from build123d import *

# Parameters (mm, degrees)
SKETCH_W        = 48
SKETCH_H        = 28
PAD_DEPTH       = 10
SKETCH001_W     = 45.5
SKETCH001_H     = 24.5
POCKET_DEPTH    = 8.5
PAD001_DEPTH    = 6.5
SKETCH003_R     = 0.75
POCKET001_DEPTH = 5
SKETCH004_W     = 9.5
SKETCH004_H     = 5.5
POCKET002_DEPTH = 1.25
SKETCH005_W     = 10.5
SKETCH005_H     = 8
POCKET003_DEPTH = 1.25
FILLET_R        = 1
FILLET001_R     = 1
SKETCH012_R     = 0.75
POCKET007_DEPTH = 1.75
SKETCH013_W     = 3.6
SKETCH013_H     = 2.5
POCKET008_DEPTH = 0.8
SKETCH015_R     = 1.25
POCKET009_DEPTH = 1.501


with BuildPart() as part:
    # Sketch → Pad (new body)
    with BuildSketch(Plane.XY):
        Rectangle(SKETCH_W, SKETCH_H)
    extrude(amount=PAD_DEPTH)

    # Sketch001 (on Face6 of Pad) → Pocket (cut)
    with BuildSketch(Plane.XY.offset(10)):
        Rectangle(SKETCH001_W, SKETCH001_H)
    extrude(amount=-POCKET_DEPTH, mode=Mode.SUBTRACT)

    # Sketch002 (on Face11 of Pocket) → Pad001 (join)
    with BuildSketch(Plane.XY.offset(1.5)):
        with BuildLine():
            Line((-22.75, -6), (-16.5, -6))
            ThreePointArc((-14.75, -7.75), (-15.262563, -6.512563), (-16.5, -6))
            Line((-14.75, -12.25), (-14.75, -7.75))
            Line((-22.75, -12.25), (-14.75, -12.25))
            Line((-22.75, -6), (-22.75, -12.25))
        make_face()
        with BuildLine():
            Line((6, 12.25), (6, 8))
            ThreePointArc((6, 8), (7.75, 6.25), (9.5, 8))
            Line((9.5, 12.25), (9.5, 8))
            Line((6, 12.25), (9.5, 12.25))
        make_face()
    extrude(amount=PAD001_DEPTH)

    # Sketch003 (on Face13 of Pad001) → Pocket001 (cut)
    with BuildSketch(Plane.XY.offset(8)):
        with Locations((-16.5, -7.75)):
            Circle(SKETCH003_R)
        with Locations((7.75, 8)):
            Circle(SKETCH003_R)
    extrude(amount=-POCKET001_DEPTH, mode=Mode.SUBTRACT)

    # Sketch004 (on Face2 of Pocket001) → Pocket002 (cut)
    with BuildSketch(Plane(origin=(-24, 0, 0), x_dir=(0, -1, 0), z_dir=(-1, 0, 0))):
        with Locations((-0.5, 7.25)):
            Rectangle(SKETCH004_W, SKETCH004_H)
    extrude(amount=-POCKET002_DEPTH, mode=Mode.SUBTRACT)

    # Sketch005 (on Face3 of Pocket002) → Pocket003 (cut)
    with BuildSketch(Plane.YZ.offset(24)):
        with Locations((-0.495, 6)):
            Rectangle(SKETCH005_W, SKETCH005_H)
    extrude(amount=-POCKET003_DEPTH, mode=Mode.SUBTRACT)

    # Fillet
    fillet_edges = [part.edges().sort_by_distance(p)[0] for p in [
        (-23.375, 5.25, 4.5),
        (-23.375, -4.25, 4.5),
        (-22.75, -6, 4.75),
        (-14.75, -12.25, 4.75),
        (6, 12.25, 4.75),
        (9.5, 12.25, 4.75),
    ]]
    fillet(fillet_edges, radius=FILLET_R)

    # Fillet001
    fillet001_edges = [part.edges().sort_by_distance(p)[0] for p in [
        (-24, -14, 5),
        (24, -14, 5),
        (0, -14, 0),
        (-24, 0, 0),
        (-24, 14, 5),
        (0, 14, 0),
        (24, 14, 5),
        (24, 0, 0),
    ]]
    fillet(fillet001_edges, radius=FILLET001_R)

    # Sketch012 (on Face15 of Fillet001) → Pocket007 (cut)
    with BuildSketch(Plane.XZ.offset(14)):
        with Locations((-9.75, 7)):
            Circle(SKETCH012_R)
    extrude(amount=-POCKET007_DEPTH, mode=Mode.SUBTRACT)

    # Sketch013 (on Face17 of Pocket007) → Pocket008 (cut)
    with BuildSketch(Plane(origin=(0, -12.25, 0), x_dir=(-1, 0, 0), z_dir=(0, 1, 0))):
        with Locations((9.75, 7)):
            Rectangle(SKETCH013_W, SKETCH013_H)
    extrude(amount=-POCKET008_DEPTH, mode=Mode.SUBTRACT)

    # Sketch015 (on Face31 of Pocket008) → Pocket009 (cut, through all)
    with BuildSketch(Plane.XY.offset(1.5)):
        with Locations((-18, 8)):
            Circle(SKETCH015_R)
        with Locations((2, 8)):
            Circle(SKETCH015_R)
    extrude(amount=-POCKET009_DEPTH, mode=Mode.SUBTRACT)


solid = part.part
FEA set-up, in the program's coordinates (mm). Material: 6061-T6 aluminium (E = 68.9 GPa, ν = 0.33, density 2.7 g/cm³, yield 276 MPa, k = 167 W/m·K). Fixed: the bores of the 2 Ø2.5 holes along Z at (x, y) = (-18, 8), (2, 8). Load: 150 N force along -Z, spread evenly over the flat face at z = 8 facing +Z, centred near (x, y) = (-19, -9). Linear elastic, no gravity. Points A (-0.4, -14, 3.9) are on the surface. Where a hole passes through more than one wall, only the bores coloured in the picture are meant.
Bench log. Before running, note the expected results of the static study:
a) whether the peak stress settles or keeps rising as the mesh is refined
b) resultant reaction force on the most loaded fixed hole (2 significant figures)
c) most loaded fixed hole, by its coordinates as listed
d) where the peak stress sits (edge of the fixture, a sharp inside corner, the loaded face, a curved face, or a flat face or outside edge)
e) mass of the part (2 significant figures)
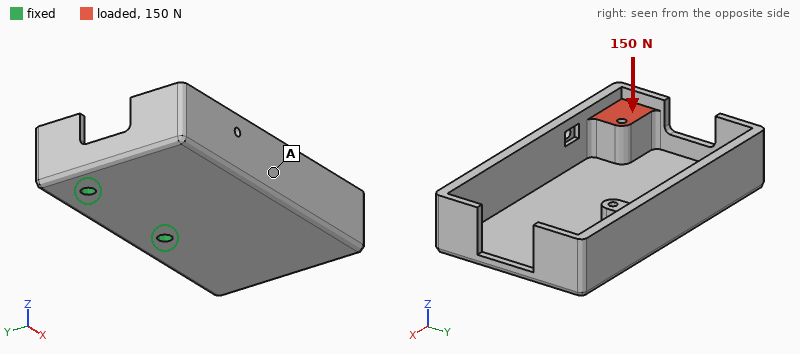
keeps rising
140 N
(-18, 8)
edge of the fixture
11 g
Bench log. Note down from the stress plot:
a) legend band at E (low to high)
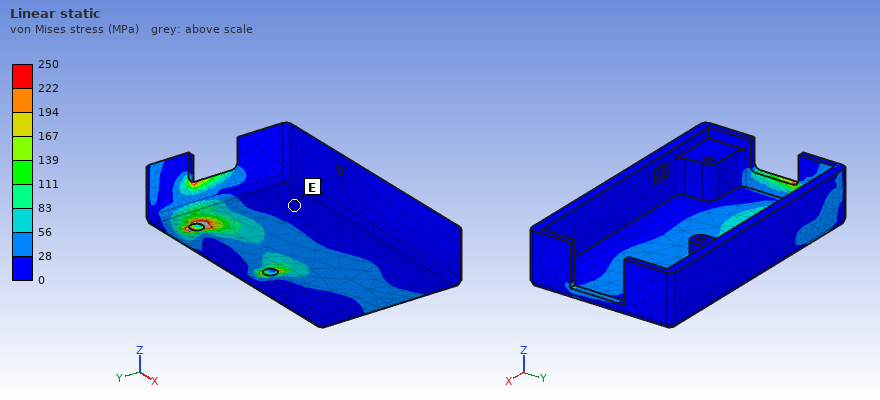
0 to 28 MPa
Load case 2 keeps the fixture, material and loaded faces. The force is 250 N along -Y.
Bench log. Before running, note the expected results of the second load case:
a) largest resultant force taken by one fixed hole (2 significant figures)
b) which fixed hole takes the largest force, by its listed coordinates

250 N
(-18, 8)
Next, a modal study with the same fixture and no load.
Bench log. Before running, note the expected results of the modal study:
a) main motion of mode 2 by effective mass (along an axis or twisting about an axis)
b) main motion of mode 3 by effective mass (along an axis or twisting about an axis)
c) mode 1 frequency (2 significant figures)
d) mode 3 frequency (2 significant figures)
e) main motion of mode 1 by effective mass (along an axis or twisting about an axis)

twisting about Y
along Z
1500 Hz
5500 Hz
along Z
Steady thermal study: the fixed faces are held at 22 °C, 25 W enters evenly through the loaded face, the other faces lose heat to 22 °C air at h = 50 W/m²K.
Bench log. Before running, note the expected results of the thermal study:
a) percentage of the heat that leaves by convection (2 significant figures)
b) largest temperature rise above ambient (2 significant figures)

21 %
70 K
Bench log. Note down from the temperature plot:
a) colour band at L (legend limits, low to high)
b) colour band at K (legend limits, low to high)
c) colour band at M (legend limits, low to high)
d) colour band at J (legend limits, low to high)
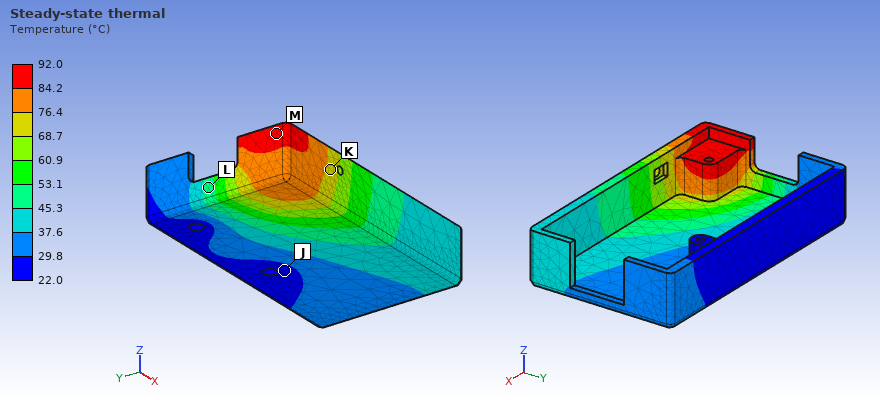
45.3 to 53.1 °C
68.7 to 76.4 °C
84.2 to 92.0 °C
22.0 to 29.8 °C
